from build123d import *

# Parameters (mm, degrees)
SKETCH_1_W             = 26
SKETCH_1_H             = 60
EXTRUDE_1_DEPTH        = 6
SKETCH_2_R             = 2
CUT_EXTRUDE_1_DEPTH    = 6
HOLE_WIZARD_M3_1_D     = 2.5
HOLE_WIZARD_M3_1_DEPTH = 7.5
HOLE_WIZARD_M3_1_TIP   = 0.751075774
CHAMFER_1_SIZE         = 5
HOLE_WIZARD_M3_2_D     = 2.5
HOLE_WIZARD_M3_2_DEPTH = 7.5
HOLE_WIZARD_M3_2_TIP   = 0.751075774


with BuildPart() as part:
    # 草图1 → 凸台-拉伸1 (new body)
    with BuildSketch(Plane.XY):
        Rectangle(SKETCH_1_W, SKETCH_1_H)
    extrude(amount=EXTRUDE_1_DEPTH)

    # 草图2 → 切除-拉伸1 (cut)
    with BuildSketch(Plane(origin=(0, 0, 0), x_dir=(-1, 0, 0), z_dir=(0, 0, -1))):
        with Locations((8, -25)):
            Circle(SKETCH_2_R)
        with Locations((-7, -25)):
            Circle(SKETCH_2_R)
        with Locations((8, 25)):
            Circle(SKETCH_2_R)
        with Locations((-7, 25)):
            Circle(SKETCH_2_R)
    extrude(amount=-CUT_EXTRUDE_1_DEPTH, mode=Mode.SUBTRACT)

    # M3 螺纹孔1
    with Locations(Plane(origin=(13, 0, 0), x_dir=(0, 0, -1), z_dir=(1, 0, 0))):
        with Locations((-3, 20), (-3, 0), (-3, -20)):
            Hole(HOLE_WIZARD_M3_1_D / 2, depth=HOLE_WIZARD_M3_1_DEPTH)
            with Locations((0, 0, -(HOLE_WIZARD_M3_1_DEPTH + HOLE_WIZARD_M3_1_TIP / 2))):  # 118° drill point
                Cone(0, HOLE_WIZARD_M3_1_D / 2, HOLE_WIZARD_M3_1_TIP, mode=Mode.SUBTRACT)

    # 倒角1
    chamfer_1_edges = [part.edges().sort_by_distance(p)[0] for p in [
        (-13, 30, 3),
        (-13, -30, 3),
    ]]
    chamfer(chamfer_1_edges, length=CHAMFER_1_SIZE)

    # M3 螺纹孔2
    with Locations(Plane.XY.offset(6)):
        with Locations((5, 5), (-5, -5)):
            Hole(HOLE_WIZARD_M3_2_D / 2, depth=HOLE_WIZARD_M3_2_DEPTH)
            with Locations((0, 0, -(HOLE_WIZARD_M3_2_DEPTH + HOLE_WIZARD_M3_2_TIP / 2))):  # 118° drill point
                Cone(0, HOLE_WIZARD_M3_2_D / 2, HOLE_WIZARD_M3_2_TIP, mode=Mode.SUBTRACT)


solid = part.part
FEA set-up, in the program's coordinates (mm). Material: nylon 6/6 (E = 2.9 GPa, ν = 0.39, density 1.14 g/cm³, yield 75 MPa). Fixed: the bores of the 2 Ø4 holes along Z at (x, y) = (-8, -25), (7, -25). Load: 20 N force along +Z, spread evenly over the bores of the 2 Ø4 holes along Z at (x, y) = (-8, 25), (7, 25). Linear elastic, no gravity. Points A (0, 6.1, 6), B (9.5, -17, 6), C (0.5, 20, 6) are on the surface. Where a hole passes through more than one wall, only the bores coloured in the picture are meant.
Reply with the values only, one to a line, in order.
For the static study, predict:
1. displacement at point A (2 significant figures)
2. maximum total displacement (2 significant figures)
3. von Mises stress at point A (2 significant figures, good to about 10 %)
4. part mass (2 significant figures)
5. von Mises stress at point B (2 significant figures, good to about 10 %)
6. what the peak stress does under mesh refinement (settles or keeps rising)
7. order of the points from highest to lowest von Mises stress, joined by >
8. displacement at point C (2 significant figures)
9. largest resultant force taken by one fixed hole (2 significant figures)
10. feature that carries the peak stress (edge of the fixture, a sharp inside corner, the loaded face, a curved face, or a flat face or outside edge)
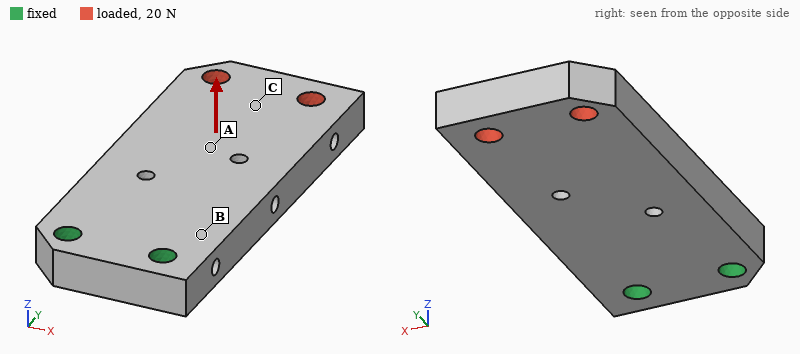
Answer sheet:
0.28 mm
0.70 mm
2.5 MPa
10.0 g
5.4 MPa
keeps rising
B > A > C
0.52 mm
10 N
edge of the fixture
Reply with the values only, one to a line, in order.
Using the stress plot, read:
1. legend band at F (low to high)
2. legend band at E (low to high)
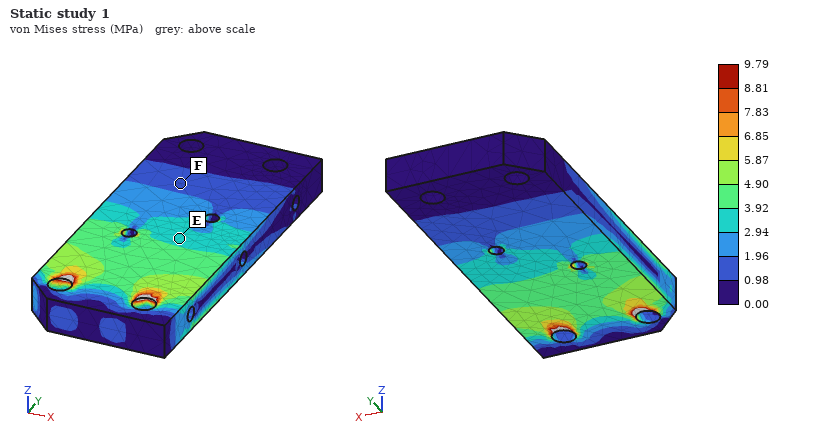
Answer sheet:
0.98 to 1.96 MPa
2.94 to 3.92 MPa
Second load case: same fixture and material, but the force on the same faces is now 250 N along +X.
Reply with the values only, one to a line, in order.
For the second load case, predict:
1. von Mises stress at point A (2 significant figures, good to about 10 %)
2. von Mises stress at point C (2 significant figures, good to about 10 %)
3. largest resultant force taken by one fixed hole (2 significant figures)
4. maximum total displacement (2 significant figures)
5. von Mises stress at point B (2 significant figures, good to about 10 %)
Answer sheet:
4.8 MPa
3.8 MPa
730 N
0.66 mm
15 MPa
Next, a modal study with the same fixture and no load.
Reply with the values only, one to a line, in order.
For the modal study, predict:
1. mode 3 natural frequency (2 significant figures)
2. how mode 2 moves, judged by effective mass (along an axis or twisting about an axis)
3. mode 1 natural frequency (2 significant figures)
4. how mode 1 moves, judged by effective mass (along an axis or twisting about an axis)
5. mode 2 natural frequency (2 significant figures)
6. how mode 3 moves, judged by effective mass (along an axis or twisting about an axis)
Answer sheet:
2100 Hz
along X
540 Hz
along Z
1900 Hz
twisting about Y
